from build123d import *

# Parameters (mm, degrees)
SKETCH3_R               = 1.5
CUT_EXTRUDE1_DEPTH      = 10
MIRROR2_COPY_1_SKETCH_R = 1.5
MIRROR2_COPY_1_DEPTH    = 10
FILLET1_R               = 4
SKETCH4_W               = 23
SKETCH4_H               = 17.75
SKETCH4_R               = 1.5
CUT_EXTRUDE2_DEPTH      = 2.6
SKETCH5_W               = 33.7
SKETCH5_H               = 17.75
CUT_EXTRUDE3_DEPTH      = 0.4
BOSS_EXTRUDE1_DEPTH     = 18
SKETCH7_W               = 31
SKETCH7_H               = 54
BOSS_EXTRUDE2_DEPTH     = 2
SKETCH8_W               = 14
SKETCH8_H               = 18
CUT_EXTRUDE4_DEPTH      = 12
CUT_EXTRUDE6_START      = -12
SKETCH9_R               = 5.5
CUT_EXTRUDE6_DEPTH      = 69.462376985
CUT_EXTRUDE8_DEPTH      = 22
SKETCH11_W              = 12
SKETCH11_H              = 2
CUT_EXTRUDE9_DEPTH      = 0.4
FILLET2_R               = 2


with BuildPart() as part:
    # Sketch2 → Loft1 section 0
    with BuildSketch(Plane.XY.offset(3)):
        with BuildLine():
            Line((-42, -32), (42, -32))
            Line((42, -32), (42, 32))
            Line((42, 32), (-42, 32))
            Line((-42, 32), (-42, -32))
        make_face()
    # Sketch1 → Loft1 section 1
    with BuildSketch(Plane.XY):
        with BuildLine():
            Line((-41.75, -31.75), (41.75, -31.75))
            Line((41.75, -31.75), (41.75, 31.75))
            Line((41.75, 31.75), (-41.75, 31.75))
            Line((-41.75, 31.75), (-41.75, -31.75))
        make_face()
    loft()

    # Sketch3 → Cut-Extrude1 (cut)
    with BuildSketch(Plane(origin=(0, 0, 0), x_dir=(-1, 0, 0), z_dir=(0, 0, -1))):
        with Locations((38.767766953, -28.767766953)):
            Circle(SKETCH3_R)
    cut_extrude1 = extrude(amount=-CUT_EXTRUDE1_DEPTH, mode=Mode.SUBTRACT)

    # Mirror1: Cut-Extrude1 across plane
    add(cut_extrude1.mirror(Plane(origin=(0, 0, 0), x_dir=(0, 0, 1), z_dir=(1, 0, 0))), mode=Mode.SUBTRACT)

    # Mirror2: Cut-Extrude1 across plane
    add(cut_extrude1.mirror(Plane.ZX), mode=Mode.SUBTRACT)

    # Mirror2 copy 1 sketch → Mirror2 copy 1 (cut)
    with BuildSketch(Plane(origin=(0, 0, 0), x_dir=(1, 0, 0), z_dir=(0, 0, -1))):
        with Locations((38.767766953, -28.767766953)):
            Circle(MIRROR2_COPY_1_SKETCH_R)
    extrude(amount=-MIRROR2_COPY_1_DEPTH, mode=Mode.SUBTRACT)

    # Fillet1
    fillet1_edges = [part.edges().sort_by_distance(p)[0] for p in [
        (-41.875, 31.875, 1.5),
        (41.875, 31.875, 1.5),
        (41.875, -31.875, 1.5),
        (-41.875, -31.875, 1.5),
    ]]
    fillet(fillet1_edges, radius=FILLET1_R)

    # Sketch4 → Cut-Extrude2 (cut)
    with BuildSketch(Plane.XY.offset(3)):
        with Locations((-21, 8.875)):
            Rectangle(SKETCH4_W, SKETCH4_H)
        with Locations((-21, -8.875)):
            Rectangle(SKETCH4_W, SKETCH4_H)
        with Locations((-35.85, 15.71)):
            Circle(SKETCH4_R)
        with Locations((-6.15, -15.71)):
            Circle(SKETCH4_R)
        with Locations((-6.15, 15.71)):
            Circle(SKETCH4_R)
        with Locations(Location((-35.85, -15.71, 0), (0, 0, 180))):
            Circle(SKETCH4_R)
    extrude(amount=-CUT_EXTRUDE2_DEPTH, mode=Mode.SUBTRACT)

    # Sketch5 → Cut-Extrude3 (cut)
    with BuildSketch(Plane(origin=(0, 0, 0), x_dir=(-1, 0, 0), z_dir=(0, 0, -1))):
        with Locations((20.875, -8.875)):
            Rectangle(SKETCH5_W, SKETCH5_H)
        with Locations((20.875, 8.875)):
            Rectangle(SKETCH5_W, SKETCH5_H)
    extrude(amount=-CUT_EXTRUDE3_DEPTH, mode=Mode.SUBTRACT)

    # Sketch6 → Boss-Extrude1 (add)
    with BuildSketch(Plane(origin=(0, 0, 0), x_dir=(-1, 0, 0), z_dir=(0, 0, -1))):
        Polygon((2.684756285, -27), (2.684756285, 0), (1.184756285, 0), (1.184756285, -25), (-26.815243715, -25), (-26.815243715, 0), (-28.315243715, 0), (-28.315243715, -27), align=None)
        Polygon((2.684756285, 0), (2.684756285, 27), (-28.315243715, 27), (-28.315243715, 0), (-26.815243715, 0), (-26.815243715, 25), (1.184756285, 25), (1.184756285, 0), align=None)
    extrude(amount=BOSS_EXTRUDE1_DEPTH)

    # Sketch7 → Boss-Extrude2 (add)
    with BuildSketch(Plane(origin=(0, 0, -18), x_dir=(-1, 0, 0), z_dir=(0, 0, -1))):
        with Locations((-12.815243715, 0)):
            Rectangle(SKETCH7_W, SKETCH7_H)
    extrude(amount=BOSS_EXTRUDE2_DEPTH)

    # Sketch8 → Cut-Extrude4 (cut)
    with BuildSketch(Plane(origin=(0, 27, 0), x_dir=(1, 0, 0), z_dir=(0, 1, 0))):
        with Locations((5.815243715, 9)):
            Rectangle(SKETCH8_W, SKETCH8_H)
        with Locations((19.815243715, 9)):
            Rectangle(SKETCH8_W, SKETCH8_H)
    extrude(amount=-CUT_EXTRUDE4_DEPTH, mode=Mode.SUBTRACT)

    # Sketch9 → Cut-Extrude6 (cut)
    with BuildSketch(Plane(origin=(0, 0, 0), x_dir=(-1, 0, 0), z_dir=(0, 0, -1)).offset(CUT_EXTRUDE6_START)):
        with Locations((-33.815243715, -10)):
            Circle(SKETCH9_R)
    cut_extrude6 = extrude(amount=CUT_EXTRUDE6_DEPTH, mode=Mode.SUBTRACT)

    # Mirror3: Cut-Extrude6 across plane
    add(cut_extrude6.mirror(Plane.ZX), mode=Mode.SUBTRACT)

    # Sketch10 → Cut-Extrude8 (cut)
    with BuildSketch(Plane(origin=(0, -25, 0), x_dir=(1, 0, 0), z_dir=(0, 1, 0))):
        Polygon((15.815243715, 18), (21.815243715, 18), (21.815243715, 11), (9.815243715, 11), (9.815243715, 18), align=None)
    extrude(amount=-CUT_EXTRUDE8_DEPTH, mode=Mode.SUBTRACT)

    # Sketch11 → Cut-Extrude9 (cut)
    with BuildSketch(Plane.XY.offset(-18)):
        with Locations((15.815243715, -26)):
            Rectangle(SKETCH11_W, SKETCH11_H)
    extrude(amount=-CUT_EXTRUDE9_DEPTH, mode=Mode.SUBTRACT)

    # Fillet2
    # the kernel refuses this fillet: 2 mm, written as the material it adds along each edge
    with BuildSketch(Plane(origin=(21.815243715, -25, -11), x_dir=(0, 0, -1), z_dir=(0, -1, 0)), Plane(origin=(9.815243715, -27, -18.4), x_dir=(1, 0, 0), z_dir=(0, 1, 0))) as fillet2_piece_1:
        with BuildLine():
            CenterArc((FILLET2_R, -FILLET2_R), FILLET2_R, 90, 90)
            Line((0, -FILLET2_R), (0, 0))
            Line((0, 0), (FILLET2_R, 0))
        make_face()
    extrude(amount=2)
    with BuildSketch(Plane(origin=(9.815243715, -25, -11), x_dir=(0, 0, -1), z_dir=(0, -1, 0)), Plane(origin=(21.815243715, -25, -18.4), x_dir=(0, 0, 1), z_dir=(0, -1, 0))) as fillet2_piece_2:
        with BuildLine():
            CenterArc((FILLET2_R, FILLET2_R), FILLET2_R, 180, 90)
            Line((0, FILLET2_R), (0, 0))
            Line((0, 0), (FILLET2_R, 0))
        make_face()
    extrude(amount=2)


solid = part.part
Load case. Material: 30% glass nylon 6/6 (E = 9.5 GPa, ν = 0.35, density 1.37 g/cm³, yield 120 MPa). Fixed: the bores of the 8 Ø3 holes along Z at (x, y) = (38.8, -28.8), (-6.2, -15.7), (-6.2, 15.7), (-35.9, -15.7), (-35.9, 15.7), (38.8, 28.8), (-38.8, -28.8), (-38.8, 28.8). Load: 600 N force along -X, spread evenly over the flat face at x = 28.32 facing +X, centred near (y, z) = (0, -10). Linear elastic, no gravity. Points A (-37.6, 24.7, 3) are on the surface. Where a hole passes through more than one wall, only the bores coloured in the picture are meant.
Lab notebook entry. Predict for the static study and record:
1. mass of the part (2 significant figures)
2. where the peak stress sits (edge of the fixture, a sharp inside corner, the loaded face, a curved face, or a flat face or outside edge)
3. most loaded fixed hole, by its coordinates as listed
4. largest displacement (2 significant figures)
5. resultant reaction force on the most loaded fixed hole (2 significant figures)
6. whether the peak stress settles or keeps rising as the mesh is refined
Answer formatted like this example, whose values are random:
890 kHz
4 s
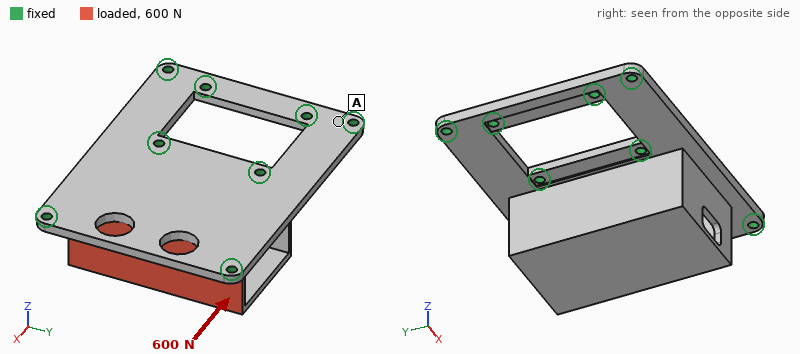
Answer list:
27 g
edge of the fixture
(-6.2, -15.7)
0.40 mm
280 N
keeps rising
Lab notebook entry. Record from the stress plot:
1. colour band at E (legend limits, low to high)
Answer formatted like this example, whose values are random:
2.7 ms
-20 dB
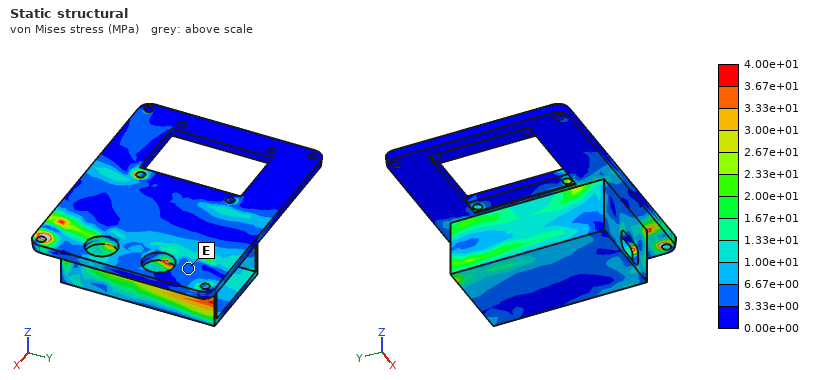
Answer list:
3.33e+00 to 6.67e+00 MPa
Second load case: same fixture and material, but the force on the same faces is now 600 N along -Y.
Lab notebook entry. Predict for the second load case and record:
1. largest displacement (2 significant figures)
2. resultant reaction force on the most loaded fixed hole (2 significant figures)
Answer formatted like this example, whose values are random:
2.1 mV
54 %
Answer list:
0.19 mm
200 N
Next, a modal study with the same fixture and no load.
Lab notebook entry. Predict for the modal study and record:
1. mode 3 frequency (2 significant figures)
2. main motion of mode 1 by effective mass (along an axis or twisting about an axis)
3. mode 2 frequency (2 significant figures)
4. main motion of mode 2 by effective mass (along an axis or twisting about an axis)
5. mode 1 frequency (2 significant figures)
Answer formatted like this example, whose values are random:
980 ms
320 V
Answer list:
3400 Hz
along X
2700 Hz
along Z
2000 Hz
